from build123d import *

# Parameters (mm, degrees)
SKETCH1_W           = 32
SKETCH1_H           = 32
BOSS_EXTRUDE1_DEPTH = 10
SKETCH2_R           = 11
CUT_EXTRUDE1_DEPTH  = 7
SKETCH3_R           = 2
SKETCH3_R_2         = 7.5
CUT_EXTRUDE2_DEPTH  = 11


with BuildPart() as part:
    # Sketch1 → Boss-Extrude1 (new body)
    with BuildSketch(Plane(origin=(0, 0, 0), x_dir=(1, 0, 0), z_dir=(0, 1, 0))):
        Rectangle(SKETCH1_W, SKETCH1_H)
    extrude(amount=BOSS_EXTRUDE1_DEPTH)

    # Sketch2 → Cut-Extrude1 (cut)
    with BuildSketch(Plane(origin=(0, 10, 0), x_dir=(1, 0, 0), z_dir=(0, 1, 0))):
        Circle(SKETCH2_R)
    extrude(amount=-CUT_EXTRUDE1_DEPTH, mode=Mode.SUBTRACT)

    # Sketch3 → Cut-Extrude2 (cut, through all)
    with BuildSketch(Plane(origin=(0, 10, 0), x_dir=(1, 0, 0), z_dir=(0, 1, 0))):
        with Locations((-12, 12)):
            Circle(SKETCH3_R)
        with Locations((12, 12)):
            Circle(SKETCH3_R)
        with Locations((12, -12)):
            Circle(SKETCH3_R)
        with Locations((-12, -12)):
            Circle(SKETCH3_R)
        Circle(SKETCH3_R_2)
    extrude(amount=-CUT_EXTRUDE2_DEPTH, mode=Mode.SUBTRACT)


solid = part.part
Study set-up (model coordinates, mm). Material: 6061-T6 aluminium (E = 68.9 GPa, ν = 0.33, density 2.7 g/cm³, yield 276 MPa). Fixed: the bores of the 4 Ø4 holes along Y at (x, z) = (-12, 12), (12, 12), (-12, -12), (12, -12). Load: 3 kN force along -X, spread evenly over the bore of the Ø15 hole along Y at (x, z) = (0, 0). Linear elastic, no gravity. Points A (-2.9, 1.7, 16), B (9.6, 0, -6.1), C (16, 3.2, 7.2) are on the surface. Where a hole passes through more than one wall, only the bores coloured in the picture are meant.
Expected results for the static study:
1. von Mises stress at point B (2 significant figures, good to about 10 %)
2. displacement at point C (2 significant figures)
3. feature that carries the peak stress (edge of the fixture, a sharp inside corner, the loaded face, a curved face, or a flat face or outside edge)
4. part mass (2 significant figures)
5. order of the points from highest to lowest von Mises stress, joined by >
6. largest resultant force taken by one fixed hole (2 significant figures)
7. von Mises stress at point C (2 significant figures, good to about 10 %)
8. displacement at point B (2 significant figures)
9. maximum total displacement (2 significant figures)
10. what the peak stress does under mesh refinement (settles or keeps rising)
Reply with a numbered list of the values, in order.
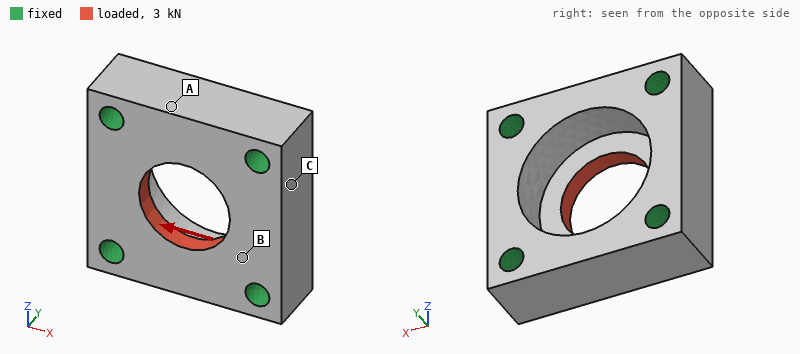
1. 26 MPa
2. 1.8 µm
3. edge of the fixture
4. 18 g
5. B > C > A
6. 780 N
7. 11 MPa
8. 2.9 µm
9. 6.4 µm
10. keeps rising
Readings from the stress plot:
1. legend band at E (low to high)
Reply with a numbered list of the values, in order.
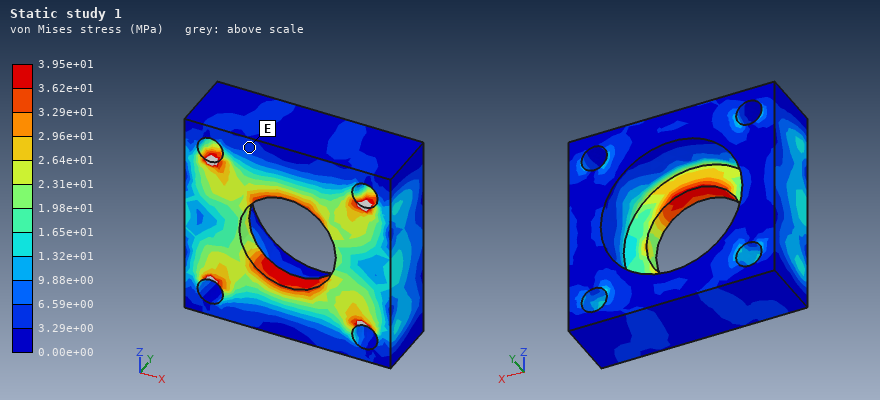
1. 3.29e+00 to 6.59e+00 MPa
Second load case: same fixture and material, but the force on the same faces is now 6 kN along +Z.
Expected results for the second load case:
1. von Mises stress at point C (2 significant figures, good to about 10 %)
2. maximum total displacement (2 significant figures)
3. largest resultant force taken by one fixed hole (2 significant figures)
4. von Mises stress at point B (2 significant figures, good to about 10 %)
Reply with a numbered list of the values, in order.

1. 7.4 MPa
2. 12 µm
3. 1.6 kN
4. 37 MPa
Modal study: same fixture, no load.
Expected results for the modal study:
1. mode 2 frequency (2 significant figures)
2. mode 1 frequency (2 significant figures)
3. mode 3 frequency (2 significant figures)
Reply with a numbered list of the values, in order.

1. 57 kHz
2. 45 kHz
3. 58 kHz
